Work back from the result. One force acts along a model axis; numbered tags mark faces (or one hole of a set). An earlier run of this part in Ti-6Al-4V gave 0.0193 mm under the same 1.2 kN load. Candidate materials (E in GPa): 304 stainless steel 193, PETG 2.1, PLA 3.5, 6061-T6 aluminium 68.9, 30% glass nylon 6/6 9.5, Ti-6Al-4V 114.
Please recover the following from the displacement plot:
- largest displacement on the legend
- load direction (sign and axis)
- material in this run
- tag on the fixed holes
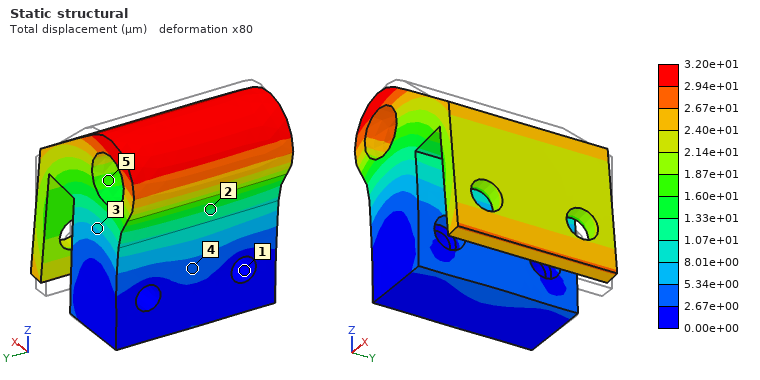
3.20e+01 µm
-X
6061-T6 aluminium
1
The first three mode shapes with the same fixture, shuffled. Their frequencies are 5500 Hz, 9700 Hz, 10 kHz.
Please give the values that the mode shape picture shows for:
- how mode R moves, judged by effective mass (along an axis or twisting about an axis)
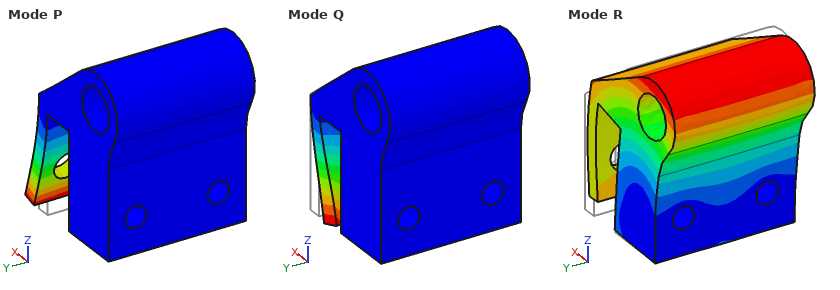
along X
